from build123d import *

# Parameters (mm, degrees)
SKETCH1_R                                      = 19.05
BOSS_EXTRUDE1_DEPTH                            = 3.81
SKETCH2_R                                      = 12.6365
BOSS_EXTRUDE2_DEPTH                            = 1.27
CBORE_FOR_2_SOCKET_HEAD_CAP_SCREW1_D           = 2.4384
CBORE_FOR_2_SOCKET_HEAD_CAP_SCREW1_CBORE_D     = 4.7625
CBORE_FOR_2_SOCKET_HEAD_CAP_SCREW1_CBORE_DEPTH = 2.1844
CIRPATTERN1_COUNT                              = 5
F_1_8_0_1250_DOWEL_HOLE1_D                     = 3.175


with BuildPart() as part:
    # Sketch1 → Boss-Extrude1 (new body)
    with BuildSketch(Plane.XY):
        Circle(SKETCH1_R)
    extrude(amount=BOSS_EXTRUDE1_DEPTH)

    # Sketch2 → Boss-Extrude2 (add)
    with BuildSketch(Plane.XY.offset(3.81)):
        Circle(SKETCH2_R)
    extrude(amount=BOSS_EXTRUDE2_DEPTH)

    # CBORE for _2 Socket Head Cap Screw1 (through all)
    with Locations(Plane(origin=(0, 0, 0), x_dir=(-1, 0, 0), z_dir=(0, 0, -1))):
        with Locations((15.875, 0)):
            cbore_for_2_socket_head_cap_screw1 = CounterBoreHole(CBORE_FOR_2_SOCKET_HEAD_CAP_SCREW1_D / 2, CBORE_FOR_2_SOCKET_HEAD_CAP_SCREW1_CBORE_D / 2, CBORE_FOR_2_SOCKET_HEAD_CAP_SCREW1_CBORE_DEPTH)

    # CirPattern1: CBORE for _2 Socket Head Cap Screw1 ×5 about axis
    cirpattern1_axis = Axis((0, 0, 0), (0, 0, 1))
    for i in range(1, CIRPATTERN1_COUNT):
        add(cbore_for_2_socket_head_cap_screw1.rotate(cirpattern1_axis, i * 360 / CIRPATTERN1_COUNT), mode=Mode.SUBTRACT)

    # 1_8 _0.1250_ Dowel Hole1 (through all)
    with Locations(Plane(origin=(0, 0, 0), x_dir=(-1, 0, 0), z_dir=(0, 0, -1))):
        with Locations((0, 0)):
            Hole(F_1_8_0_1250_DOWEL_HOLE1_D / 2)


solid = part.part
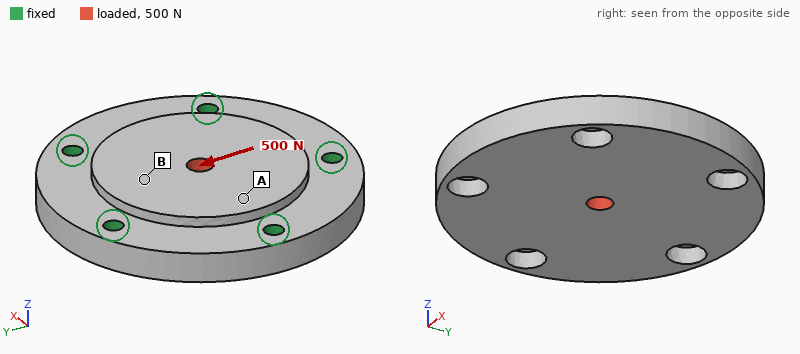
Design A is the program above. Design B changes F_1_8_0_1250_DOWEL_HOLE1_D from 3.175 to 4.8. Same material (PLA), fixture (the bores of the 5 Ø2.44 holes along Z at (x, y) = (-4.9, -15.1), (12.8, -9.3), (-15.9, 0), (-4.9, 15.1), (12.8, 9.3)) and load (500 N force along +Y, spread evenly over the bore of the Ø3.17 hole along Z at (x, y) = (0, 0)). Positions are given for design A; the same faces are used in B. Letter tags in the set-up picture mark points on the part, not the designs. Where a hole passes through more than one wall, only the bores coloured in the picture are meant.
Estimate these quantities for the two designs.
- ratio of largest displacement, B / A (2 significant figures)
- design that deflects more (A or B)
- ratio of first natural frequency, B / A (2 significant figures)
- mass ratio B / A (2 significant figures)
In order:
0.87
A
1.00
0.99
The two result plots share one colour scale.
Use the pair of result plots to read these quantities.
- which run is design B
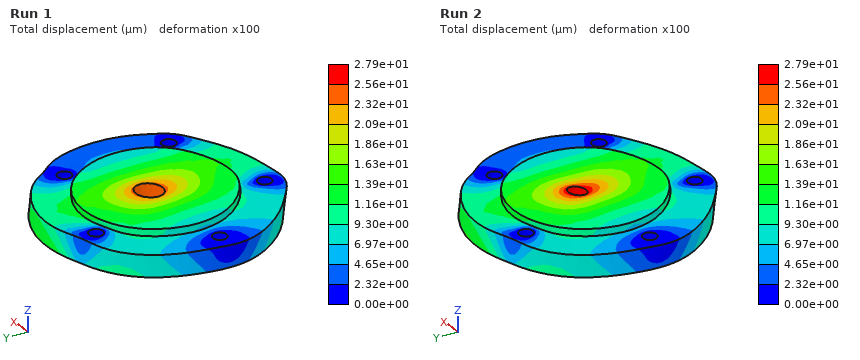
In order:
Run 1
